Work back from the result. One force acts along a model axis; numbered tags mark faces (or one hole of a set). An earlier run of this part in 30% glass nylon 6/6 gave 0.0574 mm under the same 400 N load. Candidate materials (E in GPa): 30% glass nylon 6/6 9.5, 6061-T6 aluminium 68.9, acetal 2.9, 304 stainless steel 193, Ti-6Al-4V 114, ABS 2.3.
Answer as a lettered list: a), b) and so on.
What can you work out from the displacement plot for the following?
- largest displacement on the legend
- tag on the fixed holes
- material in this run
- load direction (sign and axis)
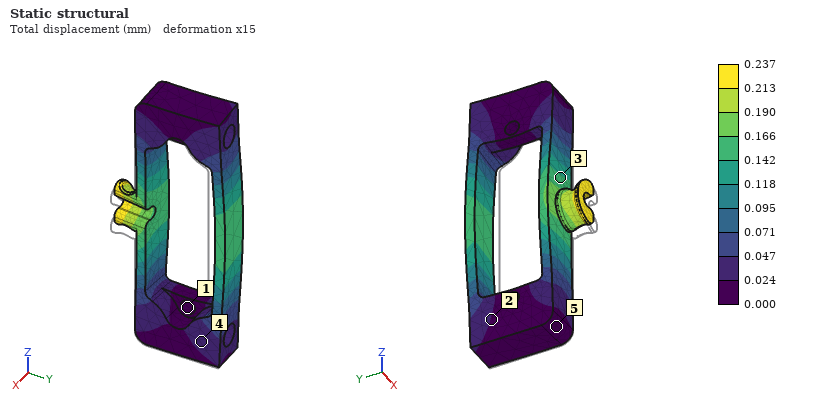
a) 0.237 mm
b) 1
c) ABS
d) -X
